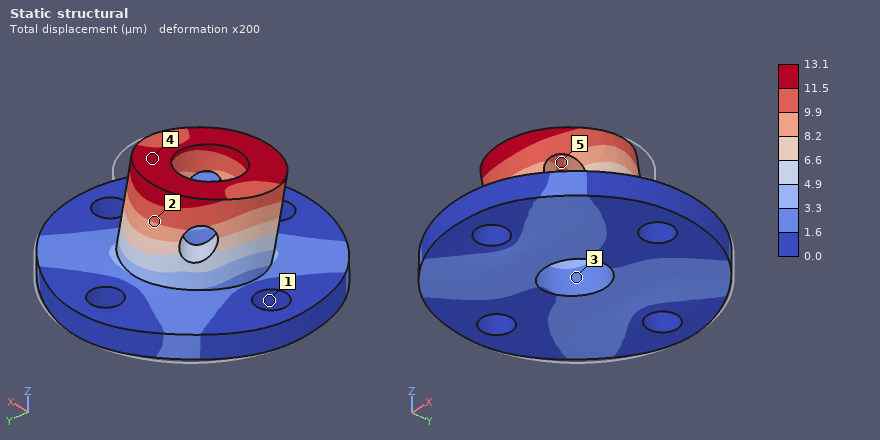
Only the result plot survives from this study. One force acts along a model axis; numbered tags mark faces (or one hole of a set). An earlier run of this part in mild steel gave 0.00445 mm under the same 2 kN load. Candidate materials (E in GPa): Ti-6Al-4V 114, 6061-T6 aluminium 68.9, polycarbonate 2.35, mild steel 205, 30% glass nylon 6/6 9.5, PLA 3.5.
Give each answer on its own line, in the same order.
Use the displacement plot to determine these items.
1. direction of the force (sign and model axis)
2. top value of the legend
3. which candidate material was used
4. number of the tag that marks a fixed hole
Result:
-Y
13.1 µm
6061-T6 aluminium
1
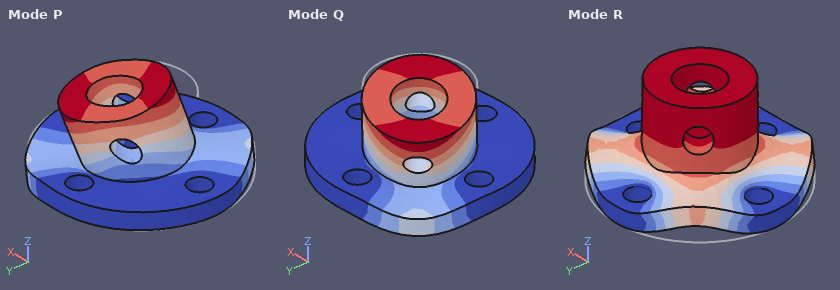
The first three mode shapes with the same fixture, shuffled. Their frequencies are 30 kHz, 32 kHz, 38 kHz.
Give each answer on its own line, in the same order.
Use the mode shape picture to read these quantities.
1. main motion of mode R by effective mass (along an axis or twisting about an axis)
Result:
along Z
